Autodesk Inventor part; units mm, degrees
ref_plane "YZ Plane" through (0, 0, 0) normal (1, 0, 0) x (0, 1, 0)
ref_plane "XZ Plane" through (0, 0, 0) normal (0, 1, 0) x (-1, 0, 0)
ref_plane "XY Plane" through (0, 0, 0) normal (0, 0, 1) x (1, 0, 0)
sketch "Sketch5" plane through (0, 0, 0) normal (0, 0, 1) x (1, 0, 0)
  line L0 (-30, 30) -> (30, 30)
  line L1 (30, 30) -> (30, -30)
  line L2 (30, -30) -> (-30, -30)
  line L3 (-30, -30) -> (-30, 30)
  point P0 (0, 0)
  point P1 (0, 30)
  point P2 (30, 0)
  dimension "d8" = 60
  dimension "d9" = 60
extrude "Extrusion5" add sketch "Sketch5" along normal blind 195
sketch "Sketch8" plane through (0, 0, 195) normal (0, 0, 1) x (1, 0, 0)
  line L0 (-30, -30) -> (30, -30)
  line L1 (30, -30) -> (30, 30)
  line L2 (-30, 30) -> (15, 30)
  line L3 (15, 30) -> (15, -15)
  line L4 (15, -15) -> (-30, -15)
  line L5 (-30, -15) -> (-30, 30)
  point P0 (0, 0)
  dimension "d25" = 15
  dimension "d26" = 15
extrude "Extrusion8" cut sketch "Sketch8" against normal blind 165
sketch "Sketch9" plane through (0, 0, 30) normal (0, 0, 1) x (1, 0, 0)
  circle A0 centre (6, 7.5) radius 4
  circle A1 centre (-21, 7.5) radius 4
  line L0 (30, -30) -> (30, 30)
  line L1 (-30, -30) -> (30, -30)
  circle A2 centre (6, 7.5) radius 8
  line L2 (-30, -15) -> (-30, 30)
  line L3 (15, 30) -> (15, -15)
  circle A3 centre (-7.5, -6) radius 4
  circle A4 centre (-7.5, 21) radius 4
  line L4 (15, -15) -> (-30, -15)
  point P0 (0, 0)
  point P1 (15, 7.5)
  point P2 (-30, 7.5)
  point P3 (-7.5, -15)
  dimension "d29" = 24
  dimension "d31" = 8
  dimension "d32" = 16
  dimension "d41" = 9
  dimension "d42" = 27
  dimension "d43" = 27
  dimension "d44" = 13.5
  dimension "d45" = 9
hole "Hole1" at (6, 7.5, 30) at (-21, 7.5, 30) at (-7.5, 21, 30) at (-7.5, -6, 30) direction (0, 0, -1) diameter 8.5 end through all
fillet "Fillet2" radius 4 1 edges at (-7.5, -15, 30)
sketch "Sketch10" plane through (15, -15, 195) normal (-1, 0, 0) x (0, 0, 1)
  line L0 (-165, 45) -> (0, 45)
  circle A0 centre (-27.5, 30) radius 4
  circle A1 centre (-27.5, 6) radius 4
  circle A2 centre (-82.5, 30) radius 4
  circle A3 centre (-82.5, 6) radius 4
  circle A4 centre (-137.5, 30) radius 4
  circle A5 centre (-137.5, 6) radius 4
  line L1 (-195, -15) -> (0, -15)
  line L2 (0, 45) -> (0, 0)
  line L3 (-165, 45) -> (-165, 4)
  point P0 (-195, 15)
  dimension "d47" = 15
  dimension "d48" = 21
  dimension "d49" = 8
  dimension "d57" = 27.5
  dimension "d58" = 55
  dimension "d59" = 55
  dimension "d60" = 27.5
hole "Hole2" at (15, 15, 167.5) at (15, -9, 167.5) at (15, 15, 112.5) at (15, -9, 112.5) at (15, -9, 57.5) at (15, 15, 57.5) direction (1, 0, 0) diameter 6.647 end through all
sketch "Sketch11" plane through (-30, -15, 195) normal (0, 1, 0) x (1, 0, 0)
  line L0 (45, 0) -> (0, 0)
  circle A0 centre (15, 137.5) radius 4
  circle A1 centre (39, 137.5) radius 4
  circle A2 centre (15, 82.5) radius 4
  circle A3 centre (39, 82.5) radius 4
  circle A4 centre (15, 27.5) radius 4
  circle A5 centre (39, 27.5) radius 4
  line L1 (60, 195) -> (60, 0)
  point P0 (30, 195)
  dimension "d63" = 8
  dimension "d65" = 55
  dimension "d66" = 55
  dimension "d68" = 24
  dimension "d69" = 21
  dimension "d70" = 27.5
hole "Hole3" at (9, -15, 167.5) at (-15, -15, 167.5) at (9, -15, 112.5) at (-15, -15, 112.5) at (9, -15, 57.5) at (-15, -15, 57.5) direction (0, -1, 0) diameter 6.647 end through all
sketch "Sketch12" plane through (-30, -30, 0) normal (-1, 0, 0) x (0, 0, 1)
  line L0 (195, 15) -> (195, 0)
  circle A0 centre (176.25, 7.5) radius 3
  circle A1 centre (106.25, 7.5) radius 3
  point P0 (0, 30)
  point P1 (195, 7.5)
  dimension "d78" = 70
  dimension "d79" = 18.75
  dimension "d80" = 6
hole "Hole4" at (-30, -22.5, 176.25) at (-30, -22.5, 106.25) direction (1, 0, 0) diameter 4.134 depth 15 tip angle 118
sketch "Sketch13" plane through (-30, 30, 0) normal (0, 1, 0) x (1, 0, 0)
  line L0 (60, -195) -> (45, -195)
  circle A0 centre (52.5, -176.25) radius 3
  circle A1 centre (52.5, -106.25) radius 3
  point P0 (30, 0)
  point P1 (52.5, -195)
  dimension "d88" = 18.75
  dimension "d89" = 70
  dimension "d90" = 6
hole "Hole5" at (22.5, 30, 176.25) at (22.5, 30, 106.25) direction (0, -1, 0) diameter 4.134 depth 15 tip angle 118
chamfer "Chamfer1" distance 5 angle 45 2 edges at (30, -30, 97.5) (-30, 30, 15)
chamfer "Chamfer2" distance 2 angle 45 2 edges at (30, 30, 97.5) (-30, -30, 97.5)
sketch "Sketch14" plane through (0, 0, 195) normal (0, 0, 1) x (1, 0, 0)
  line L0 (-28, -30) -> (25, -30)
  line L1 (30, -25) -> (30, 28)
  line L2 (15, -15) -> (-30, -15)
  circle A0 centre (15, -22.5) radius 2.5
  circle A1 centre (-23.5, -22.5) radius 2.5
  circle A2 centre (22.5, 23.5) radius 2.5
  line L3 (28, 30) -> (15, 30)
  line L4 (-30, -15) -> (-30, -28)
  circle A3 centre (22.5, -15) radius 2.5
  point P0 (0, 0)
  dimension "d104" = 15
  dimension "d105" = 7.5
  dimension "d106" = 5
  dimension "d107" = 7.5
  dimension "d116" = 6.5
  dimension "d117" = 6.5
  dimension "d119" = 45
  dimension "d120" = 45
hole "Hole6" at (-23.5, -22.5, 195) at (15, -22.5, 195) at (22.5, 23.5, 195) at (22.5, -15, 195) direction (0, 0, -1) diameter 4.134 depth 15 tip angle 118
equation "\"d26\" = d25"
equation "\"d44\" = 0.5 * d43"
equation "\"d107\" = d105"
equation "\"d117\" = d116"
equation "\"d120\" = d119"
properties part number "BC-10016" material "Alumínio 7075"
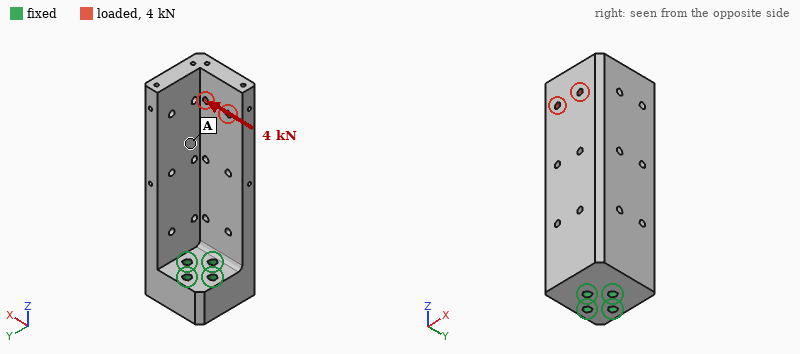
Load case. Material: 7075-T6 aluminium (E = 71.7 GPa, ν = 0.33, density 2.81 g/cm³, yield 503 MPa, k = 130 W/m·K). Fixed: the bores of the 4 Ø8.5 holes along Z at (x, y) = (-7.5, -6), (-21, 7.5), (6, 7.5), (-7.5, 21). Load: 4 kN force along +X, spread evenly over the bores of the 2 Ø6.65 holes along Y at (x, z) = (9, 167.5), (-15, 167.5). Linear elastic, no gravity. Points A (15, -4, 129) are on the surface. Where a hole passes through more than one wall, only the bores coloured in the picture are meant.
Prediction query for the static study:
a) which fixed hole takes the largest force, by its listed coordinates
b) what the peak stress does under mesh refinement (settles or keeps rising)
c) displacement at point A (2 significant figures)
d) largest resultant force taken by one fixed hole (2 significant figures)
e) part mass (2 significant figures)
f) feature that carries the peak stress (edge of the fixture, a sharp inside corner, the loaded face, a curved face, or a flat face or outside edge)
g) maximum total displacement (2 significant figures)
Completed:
(6, 7.5)
keeps rising
0.25 mm
9.1 kN
980 g
edge of the fixture
0.48 mm
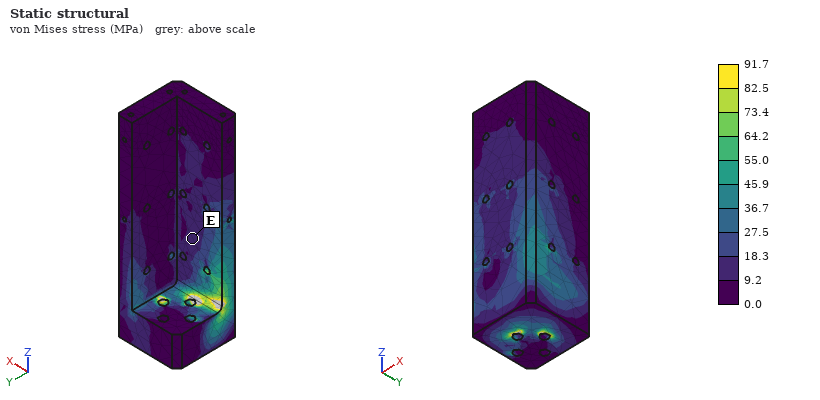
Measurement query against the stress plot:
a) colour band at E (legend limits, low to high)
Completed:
9.2 to 18.3 MPa
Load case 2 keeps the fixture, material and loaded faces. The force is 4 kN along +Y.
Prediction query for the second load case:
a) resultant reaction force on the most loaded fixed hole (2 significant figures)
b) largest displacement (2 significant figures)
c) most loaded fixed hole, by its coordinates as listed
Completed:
8.5 kN
0.70 mm
(-7.5, -6)
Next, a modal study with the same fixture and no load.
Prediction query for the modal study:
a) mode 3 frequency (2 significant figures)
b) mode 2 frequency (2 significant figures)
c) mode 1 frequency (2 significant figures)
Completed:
2100 Hz
1100 Hz
790 Hz
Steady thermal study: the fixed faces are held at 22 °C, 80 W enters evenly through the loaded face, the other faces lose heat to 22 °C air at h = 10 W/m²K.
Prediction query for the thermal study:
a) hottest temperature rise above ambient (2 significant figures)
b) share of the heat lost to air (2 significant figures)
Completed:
65 K
19 %
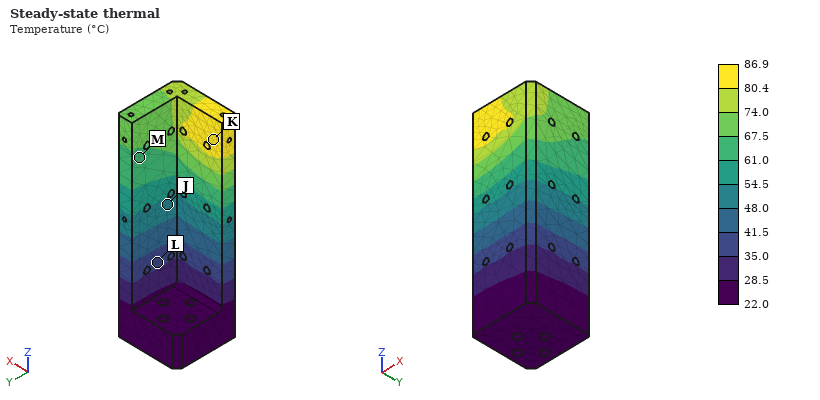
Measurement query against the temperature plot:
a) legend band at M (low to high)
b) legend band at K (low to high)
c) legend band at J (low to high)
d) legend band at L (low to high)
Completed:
61.0 to 67.5 °C
80.4 to 86.9 °C
48.0 to 54.5 °C
35.0 to 41.5 °C
